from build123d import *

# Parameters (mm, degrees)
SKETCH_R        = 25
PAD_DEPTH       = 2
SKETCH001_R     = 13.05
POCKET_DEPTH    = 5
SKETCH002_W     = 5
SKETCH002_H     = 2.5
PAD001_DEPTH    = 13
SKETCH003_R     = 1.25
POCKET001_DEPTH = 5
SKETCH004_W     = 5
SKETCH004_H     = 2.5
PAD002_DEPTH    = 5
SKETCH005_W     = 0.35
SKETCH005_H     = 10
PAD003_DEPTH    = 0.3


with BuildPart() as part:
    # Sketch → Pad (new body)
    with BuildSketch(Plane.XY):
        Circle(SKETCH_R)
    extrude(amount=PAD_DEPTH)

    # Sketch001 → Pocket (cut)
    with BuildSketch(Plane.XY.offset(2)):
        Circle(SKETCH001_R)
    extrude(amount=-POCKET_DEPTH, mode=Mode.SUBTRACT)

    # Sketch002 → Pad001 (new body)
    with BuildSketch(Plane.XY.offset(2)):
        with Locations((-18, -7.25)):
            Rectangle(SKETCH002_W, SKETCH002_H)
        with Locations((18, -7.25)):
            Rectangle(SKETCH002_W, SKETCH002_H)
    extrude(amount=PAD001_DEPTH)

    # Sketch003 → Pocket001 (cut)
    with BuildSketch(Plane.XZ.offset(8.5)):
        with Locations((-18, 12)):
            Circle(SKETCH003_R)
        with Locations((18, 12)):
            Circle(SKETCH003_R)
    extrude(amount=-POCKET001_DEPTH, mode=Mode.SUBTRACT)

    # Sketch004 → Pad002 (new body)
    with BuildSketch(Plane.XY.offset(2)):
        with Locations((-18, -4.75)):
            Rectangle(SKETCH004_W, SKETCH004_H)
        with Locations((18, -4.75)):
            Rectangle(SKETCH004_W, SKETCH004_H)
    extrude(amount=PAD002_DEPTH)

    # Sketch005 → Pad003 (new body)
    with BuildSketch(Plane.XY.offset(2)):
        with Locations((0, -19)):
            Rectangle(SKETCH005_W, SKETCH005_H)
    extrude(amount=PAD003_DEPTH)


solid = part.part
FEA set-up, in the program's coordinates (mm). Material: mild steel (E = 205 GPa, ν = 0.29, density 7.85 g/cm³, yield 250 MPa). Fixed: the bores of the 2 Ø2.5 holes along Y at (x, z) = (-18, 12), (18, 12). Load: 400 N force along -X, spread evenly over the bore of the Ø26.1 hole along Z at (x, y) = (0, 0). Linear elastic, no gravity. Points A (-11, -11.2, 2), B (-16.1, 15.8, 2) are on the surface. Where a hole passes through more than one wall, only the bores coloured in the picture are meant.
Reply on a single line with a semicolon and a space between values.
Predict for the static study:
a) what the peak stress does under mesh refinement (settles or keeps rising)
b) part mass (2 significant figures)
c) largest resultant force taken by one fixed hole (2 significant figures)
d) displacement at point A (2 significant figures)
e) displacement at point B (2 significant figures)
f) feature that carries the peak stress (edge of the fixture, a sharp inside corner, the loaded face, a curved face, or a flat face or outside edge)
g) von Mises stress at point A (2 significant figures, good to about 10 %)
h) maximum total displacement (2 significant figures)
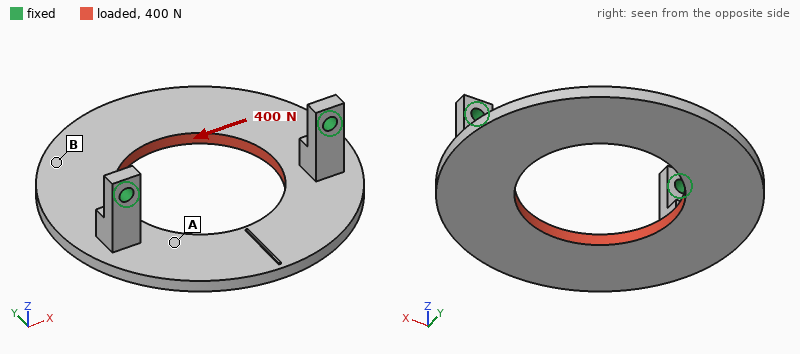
keeps rising; 26 g; 210 N; 12 µm; 31 µm; edge of the fixture; 36 MPa; 33 µm
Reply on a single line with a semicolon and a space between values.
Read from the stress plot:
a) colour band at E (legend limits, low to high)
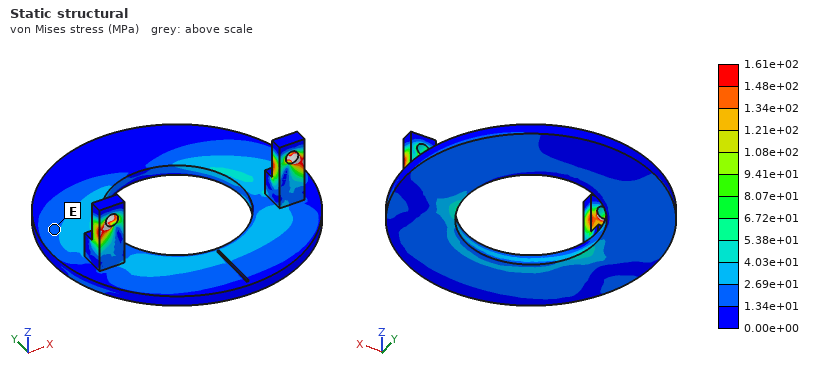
1.34e+01 to 2.69e+01 MPa
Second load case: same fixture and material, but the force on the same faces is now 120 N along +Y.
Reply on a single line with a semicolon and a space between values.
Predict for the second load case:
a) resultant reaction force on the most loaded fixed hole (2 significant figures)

60 N
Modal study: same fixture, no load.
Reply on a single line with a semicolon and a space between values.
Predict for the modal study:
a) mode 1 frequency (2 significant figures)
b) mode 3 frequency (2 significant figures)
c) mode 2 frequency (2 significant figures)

1100 Hz; 3000 Hz; 2700 Hz
